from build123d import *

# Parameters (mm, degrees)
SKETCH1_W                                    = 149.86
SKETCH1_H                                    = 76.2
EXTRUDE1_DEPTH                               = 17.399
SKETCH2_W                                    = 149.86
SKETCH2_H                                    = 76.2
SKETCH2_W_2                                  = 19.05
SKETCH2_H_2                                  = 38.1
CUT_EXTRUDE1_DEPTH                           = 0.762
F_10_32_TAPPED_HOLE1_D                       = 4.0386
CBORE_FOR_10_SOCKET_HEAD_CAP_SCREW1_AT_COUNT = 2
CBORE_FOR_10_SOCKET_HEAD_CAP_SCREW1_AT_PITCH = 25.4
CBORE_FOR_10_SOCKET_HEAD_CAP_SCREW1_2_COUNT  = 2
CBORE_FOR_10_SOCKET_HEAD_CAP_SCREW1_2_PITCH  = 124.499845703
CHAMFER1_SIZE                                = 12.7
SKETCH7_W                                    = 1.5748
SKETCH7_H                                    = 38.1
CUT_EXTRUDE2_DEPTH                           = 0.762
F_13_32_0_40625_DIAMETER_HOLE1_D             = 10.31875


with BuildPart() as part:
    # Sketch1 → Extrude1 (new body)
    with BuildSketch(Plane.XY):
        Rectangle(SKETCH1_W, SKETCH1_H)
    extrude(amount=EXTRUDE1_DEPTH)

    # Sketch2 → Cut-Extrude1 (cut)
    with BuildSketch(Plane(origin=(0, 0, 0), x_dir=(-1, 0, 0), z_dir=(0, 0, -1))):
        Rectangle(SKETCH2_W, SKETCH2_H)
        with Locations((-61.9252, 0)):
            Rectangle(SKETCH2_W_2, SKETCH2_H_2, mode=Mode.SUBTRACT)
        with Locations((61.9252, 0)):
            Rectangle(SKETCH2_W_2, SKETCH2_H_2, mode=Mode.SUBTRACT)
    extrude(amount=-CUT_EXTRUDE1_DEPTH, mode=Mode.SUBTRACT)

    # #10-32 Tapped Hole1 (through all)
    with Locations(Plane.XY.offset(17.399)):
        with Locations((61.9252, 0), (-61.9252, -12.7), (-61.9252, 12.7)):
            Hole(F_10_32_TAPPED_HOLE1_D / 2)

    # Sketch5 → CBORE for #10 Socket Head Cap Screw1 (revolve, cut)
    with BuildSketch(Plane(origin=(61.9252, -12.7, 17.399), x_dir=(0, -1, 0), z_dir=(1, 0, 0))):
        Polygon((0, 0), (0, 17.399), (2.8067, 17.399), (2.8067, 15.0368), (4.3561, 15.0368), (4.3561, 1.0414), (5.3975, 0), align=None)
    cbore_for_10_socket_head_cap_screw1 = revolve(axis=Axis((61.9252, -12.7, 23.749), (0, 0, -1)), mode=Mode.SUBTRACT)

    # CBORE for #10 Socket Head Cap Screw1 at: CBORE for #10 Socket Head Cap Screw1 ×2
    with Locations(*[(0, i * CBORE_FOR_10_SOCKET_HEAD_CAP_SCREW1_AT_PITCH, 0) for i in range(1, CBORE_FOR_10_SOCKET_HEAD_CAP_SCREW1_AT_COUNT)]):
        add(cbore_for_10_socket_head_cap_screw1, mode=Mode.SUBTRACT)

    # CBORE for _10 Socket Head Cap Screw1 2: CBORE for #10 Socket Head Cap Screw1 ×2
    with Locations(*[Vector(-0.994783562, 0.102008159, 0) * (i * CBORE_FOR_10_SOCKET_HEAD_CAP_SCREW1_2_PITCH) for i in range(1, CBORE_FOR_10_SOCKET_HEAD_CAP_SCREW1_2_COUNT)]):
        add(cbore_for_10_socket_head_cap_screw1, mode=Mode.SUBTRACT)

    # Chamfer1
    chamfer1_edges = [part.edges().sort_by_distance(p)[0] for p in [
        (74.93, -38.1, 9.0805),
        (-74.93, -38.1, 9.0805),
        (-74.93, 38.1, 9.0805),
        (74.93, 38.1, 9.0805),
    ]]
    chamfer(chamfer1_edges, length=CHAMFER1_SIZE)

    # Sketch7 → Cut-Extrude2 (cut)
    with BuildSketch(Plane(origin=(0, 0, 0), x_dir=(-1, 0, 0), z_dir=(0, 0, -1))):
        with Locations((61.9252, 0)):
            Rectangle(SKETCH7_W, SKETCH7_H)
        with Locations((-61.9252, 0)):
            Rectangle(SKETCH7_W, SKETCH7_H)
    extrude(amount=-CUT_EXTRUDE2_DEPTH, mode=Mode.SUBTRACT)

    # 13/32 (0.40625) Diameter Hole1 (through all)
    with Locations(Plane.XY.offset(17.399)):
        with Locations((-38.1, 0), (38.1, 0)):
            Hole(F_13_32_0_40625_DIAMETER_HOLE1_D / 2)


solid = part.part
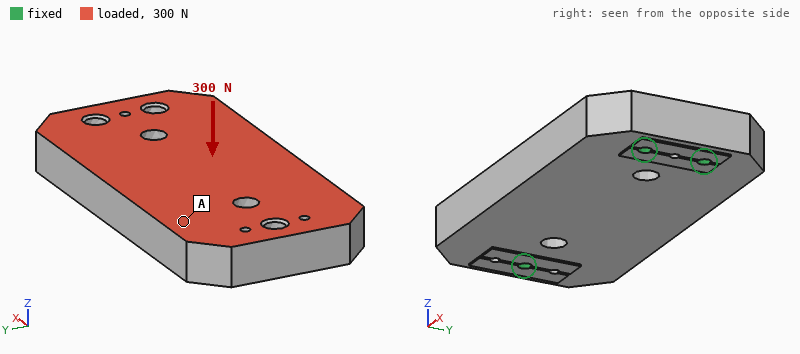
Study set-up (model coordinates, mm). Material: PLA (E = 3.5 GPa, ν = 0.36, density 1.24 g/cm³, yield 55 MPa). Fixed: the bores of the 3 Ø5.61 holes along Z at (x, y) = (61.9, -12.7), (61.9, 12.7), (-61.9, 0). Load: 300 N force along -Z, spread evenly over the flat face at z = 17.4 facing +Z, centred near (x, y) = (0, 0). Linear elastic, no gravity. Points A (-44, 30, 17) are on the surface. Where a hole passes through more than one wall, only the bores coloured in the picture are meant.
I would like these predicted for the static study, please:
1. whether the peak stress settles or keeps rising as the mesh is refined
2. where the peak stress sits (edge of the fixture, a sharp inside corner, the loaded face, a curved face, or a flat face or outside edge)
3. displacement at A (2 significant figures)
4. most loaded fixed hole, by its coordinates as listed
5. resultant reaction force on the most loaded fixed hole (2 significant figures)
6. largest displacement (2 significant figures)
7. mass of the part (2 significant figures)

keeps rising
edge of the fixture
31 µm
(-61.9, 0)
210 N
51 µm
220 g
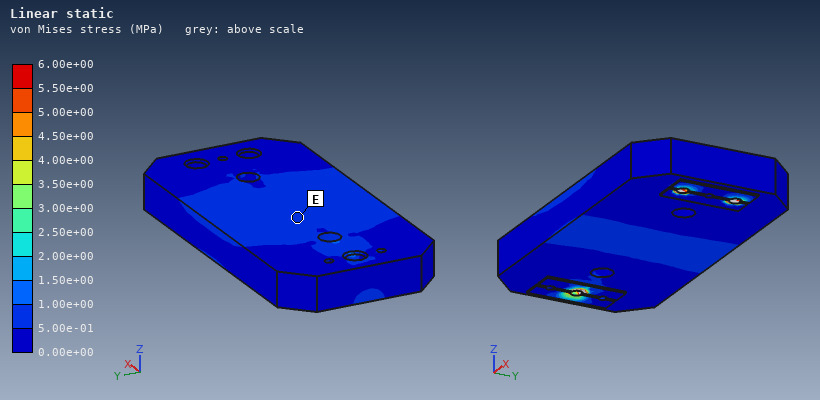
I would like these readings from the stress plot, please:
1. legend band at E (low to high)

5.00e-01 to 1.00e+00 MPa
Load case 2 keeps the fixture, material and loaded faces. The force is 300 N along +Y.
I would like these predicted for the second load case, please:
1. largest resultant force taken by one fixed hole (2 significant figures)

200 N
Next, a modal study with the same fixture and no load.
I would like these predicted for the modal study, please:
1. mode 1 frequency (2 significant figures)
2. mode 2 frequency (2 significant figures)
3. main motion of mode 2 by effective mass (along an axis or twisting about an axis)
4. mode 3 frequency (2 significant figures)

660 Hz
950 Hz
along Z
1900 Hz
